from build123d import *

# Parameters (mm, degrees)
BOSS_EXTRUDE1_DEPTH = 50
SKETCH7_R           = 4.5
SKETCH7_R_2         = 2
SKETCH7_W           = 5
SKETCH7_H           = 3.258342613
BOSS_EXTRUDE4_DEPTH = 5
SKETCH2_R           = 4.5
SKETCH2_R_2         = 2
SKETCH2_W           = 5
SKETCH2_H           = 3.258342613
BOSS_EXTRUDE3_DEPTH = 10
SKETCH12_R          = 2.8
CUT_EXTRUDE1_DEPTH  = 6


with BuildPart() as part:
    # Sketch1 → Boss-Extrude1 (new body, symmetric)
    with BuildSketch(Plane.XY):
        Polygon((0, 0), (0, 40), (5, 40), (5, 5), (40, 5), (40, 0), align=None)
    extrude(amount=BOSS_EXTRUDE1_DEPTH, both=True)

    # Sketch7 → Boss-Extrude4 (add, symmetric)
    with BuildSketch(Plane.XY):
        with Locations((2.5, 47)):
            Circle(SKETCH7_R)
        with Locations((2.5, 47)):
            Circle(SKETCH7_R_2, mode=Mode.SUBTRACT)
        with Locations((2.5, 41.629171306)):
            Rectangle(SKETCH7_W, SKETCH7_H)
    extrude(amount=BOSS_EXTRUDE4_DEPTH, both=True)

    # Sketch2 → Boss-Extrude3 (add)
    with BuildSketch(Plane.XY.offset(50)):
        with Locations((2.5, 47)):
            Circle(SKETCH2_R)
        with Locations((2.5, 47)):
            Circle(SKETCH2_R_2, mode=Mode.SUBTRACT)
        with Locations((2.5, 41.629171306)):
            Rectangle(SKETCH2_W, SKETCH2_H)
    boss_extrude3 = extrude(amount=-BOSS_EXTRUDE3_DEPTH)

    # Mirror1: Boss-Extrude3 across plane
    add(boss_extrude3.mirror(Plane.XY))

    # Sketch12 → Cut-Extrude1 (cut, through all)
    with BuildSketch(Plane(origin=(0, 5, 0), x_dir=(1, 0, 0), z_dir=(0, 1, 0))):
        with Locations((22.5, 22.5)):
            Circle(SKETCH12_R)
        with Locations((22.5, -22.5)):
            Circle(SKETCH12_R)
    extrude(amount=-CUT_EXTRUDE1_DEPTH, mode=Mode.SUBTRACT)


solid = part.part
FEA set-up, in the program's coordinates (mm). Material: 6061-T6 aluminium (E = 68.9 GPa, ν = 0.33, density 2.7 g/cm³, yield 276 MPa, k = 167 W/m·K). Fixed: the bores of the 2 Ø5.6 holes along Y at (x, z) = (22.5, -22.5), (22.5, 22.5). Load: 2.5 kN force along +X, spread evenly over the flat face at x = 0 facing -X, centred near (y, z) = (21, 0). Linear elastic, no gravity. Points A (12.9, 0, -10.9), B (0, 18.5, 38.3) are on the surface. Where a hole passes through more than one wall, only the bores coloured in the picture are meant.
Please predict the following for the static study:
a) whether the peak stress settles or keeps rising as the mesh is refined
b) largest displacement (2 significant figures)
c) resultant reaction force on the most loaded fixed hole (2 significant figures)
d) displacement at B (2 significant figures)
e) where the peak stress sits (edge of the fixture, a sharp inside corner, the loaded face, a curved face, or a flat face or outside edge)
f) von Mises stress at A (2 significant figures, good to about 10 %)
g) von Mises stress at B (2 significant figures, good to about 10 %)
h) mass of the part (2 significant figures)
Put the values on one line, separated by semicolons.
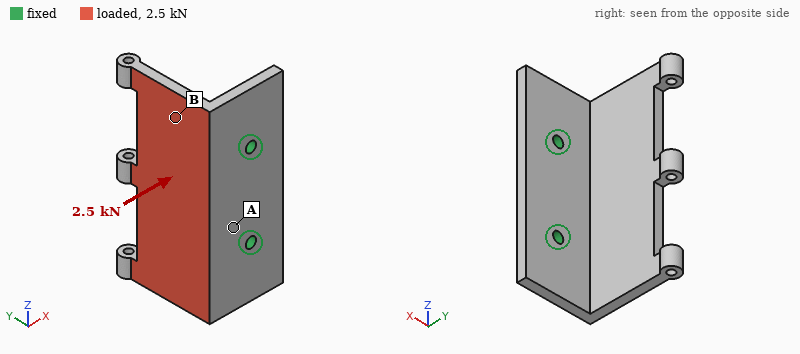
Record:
keeps rising; 0.94 mm; 1.3 kN; 0.33 mm; edge of the fixture; 94 MPa; 32 MPa; 110 g
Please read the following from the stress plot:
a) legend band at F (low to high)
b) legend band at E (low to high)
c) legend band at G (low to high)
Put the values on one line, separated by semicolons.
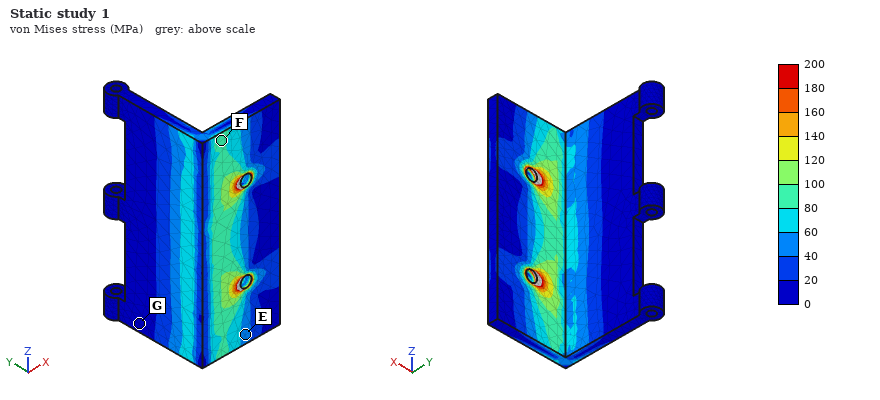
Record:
80 to 100 MPa; 40 to 60 MPa; 0 to 20 MPa
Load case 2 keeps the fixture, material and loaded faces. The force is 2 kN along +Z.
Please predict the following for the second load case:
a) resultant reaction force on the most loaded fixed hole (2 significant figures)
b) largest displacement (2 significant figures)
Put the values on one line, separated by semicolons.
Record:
1.5 kN; 0.13 mm
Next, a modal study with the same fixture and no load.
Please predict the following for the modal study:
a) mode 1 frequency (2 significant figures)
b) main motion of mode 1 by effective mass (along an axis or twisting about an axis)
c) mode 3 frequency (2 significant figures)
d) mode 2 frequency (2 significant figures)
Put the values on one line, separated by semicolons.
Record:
1300 Hz; along X; 3000 Hz; 1900 Hz
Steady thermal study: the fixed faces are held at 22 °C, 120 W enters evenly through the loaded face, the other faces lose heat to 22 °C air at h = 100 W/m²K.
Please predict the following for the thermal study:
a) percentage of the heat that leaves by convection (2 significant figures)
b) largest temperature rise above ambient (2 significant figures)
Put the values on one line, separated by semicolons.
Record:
30 %; 47 K
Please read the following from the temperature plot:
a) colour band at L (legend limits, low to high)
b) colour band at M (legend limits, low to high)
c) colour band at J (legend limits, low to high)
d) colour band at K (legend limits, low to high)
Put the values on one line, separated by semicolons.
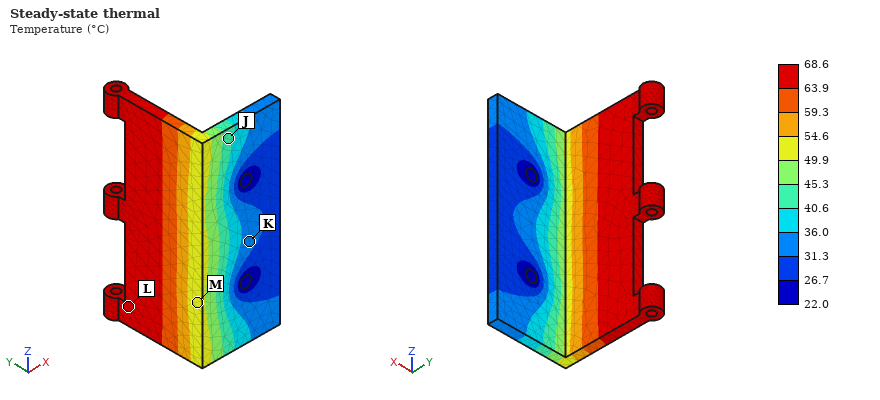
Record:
63.9 to 68.6 °C; 49.9 to 54.6 °C; 40.6 to 45.3 °C; 31.3 to 36.0 °C
